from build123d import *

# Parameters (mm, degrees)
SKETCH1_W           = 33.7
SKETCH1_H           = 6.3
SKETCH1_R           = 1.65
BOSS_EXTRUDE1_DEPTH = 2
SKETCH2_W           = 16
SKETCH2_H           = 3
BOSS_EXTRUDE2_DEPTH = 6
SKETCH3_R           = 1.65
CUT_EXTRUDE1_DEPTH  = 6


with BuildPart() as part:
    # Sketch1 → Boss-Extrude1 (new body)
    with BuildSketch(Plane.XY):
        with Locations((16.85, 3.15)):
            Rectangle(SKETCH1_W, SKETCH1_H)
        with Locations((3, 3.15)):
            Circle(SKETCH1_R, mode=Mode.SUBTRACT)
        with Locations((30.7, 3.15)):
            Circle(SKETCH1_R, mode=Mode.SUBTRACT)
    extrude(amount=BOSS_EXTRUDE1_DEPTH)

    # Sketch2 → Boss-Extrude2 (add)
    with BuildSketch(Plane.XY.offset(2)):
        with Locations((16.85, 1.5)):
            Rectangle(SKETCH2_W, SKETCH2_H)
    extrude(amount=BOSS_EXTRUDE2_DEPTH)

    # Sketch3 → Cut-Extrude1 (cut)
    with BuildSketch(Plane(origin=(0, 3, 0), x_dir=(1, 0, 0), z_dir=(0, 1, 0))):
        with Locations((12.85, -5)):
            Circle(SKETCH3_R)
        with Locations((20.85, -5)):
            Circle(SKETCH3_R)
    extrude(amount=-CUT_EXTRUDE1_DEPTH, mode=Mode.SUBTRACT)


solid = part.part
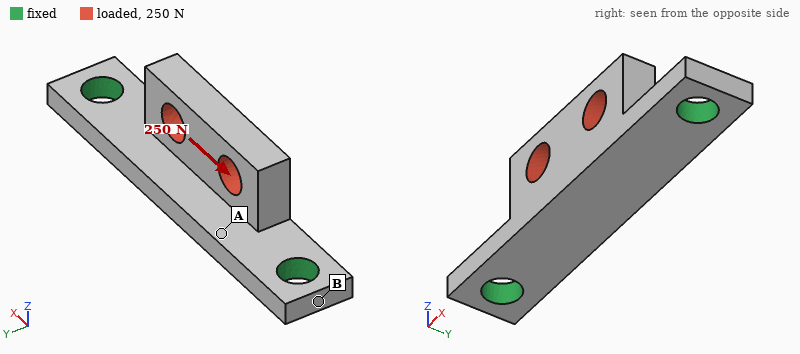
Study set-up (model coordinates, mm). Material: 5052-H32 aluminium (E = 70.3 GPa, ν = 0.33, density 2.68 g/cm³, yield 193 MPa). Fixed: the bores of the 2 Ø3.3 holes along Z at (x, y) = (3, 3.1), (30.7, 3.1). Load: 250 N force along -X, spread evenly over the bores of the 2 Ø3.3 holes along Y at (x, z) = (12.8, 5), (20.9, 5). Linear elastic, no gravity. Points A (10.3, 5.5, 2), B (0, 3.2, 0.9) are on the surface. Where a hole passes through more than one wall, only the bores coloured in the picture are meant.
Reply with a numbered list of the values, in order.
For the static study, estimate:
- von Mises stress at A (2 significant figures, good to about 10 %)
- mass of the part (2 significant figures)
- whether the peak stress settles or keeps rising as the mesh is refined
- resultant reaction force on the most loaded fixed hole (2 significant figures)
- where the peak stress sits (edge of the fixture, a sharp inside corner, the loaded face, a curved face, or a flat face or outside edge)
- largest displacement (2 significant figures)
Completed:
1. 15 MPa
2. 1.7 g
3. keeps rising
4. 140 N
5. edge of the fixture
6. 7.0 µm
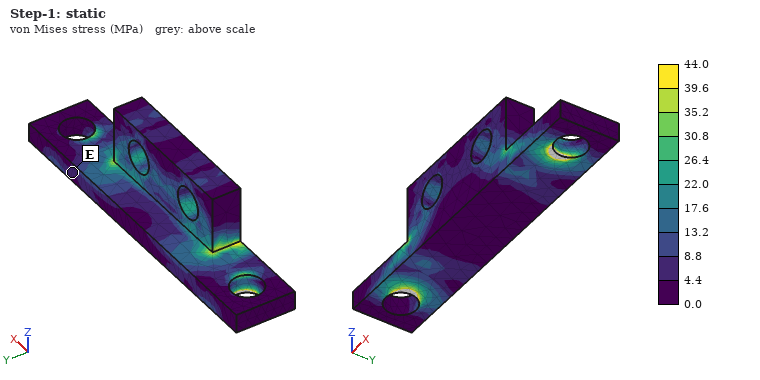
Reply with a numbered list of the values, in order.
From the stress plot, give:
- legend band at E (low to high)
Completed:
1. 4.4 to 8.8 MPa
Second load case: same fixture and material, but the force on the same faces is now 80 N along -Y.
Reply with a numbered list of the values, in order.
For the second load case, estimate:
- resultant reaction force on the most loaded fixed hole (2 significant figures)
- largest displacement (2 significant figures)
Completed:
1. 40 N
2. 23 µm
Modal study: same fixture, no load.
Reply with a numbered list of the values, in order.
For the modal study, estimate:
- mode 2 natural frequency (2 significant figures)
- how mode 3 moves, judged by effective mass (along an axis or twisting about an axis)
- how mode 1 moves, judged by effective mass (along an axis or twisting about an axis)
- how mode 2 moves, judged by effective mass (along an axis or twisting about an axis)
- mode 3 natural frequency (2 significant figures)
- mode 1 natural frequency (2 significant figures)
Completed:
1. 19 kHz
2. along Y
3. along Y
4. along Z
5. 32 kHz
6. 13 kHz
